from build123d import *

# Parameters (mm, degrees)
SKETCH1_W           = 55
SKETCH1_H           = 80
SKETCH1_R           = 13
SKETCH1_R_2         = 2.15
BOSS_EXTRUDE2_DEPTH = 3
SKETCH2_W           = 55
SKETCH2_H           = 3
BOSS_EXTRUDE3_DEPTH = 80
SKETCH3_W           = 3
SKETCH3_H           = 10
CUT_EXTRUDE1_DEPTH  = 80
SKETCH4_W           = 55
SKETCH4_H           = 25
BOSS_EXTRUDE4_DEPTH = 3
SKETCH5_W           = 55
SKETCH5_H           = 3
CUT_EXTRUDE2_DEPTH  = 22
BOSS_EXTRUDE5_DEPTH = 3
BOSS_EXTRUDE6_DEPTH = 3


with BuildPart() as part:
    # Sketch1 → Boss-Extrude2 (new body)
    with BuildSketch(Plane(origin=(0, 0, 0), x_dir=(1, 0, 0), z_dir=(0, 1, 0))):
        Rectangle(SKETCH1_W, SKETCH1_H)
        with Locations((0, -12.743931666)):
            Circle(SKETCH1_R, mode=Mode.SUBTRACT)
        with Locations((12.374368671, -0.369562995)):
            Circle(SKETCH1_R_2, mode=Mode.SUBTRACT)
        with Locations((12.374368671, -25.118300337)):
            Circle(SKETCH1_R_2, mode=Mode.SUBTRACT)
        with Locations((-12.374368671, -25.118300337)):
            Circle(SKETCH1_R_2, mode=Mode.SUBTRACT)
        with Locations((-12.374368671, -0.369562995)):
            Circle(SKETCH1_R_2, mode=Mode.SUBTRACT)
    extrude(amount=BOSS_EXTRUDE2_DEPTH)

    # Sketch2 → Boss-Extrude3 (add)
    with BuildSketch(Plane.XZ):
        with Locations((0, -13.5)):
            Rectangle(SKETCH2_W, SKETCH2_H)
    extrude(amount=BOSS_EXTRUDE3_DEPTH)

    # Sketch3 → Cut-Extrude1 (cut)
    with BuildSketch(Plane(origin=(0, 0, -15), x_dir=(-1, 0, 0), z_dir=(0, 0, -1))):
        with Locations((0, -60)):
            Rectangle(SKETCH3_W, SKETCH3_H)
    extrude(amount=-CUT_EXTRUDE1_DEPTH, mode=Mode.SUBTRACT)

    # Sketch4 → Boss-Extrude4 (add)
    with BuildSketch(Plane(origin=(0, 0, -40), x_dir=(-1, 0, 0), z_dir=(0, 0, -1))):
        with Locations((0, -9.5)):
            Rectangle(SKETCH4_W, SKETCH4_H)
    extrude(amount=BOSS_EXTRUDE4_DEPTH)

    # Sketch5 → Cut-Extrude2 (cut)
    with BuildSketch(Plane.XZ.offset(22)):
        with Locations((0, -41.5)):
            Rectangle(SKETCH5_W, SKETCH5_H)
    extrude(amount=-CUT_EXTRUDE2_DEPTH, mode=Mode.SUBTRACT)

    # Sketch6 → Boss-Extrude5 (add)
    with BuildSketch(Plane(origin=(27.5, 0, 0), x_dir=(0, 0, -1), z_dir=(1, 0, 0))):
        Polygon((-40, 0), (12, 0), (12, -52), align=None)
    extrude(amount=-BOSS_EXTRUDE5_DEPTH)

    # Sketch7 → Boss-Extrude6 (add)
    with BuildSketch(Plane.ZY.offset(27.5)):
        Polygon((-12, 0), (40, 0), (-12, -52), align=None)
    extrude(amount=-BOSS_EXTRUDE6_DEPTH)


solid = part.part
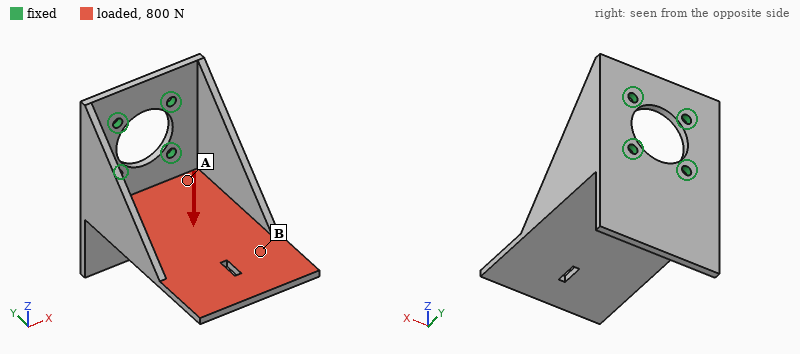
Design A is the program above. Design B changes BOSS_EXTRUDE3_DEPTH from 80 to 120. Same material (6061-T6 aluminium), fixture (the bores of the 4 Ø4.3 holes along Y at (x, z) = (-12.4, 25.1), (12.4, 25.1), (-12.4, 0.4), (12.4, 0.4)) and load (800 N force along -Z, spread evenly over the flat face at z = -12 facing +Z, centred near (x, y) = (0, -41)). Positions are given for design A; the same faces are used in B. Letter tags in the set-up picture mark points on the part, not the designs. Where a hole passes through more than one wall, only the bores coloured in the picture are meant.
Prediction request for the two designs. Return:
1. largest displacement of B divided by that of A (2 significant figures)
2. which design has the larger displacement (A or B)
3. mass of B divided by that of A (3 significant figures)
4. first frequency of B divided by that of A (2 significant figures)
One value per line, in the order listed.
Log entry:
6.0
B
1.20
0.34
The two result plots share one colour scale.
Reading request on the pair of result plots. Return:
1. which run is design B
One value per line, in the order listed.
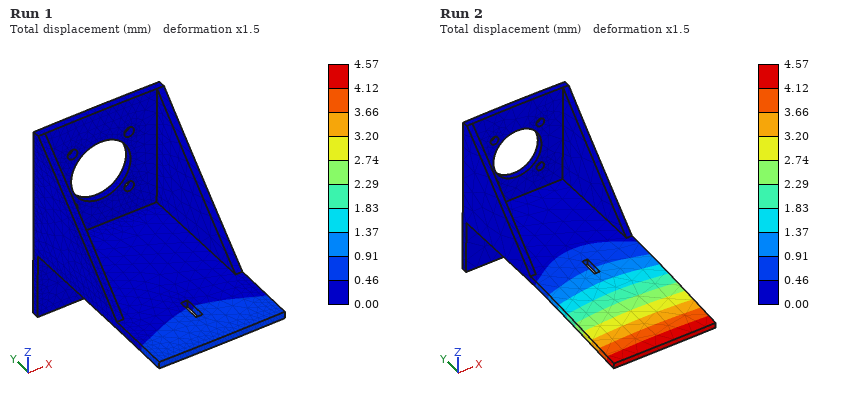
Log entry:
Run 2
